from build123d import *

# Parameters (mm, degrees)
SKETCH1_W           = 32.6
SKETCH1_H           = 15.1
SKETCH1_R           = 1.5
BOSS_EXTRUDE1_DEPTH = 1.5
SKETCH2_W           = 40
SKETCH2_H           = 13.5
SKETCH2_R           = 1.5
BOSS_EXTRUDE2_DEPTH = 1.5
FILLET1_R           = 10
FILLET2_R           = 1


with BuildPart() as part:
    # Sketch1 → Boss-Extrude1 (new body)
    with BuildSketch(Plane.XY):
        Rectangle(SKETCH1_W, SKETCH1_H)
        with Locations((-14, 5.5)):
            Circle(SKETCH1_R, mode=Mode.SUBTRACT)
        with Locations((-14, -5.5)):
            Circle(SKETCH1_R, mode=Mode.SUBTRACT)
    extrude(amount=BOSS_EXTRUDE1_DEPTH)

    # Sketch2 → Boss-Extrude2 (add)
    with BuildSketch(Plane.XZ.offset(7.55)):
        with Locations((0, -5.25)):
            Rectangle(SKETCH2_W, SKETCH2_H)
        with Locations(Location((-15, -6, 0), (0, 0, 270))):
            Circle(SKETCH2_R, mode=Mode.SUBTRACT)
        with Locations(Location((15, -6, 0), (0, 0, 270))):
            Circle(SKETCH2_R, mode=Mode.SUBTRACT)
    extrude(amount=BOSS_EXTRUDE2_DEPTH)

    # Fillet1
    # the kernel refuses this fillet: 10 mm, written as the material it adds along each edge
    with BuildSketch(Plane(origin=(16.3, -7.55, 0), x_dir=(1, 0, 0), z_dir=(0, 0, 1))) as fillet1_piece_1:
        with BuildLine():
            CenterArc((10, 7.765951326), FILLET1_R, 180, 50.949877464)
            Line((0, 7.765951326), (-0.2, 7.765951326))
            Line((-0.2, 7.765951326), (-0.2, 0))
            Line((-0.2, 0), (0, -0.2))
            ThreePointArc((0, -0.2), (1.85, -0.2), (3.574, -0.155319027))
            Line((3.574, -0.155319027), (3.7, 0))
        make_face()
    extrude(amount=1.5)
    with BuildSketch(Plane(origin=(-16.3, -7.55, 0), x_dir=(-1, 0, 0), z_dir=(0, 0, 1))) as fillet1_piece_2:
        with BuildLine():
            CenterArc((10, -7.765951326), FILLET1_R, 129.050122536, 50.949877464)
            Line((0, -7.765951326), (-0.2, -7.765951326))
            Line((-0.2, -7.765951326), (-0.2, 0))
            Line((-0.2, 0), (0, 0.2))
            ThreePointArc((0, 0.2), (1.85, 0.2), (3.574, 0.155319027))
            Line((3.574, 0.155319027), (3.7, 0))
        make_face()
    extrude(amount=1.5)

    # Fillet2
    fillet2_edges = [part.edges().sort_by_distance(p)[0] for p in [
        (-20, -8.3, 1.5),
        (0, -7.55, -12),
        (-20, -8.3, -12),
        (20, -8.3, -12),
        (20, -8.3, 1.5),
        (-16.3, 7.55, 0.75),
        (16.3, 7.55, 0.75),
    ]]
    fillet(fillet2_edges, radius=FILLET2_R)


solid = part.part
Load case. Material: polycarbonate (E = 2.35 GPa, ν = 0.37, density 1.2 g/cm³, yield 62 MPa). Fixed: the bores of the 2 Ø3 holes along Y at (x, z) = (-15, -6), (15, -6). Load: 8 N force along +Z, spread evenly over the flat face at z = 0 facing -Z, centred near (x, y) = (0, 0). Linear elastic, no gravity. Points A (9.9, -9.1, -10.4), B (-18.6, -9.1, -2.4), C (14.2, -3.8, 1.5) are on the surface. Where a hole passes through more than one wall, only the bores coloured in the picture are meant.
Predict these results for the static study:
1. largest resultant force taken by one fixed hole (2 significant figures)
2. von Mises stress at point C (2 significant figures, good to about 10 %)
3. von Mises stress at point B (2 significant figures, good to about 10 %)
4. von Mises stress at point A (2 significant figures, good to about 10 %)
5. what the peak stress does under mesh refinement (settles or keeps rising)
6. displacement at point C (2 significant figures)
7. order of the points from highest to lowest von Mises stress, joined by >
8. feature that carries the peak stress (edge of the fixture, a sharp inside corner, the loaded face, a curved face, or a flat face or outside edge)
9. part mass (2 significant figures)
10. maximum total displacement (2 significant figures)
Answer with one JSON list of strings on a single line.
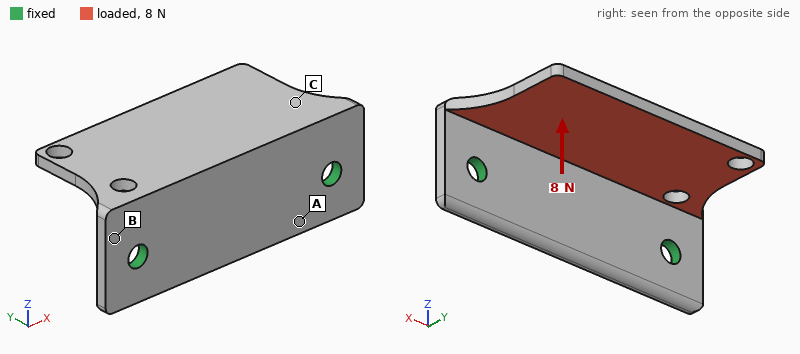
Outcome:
["4.2 N", "2.8 MPa", "4.1 MPa", "1.1 MPa", "keeps rising", "0.12 mm", "B > C > A", "edge of the fixture", "1.8 g", "0.45 mm"]
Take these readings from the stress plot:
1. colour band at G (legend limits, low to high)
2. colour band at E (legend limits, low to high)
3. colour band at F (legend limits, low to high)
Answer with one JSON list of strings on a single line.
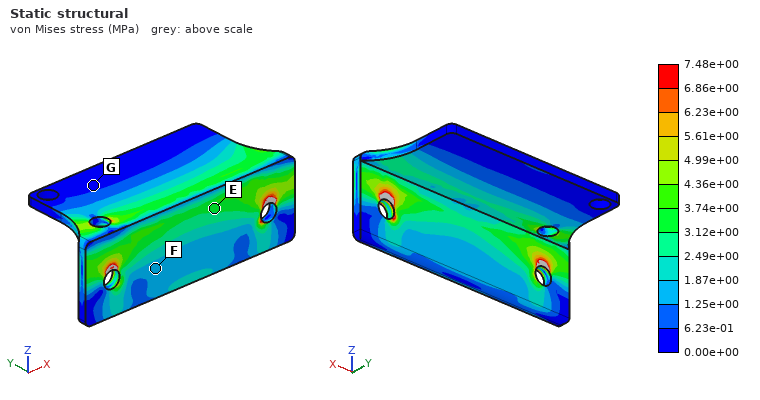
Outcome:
["0.00e+00 to 6.23e-01 MPa", "3.12e+00 to 3.74e+00 MPa", "1.25e+00 to 1.87e+00 MPa"]
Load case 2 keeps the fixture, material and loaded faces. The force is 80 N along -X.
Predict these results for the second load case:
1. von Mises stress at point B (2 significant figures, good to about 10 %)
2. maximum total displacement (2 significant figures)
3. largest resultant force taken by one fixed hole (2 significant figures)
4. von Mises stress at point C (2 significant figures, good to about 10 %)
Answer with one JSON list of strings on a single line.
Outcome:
["11 MPa", "0.50 mm", "48 N", "3.5 MPa"]
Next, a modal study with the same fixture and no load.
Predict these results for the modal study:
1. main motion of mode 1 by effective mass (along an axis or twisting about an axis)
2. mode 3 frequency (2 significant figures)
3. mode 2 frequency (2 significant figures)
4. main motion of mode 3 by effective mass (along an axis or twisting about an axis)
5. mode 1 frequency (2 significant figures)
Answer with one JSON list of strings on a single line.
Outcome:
["along Z", "2700 Hz", "1700 Hz", "along Y", "870 Hz"]
